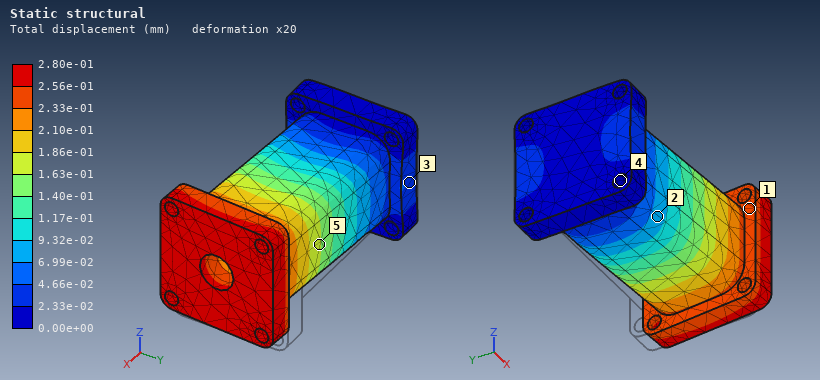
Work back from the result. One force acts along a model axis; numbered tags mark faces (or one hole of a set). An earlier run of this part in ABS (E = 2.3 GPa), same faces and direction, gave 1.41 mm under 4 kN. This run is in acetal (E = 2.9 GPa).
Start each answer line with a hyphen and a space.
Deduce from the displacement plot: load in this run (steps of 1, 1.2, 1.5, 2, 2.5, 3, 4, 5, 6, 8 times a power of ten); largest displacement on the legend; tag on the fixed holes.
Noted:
- 1 kN
- 2.80e-01 mm
- 4
